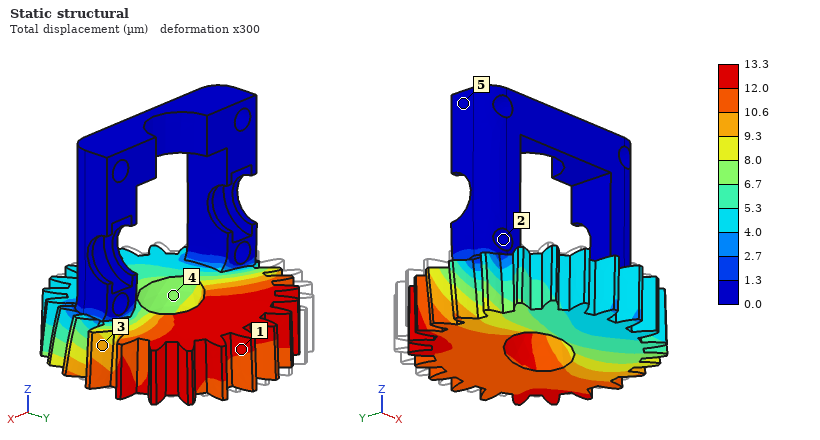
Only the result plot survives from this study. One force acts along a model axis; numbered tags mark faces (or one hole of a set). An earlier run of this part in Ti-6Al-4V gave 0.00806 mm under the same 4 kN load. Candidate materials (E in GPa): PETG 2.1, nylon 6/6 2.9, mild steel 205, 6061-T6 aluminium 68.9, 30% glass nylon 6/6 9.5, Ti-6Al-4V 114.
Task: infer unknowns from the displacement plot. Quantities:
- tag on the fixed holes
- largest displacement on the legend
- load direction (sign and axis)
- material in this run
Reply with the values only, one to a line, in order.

2
13.3 µm
+X
6061-T6 aluminium
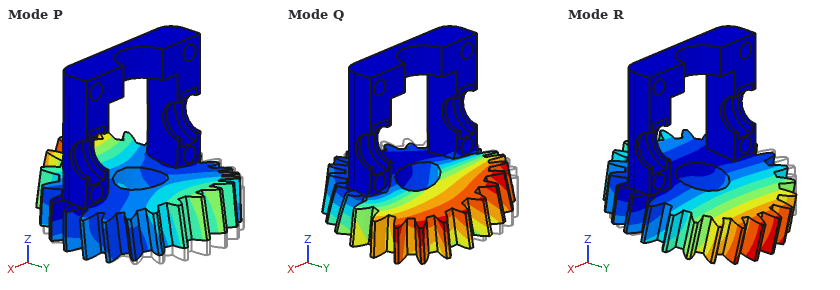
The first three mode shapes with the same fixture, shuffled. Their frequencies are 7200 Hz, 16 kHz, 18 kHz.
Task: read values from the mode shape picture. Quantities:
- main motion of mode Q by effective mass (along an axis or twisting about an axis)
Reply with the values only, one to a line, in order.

along X
